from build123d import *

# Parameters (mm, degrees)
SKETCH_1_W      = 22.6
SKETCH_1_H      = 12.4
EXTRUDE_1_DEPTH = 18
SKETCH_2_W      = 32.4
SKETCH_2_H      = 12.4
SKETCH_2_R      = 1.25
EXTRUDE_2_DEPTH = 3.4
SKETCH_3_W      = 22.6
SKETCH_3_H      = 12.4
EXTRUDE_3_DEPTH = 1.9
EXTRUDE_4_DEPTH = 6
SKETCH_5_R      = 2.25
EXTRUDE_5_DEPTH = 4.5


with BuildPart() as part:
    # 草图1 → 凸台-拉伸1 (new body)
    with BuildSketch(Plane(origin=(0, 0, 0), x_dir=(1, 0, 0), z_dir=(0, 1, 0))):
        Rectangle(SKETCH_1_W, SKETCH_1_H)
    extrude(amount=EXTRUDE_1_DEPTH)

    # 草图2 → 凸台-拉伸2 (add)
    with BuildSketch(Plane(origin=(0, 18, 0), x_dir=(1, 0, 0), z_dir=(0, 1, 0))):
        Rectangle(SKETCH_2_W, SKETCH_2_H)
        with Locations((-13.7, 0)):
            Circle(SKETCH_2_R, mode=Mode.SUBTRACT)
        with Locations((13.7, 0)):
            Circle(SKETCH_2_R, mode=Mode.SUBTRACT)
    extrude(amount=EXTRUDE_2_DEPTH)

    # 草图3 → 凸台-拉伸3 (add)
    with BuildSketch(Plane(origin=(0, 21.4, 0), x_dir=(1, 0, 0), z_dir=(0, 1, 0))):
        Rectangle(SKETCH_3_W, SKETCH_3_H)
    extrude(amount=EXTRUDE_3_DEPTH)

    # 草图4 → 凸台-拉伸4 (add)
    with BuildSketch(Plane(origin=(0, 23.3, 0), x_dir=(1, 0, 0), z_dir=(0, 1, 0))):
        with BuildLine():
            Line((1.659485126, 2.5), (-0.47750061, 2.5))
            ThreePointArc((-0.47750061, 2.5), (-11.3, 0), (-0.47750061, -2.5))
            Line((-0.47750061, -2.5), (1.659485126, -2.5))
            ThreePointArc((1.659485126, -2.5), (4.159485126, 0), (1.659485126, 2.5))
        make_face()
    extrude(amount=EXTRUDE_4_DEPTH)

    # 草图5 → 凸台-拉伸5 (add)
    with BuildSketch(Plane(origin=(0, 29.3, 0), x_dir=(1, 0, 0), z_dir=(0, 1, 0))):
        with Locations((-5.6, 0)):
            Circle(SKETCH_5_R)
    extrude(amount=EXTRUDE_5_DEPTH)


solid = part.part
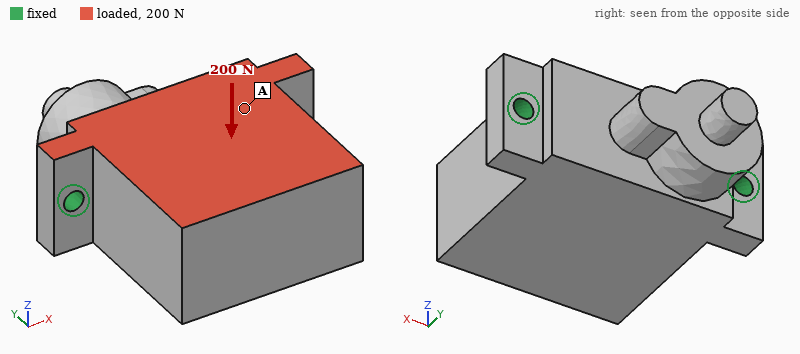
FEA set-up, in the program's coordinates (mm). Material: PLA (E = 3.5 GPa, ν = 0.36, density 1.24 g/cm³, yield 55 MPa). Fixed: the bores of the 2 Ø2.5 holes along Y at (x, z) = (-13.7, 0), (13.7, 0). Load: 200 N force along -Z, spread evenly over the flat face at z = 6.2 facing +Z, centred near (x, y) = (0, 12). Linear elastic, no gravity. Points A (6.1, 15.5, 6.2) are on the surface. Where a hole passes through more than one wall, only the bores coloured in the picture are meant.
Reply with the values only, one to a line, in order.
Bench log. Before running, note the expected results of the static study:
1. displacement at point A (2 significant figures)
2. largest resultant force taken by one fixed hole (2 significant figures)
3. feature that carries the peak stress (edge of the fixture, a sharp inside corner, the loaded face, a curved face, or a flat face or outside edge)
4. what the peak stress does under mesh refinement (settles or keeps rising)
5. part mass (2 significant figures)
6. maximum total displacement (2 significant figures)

0.11 mm
100 N
edge of the fixture
keeps rising
9.6 g
0.30 mm
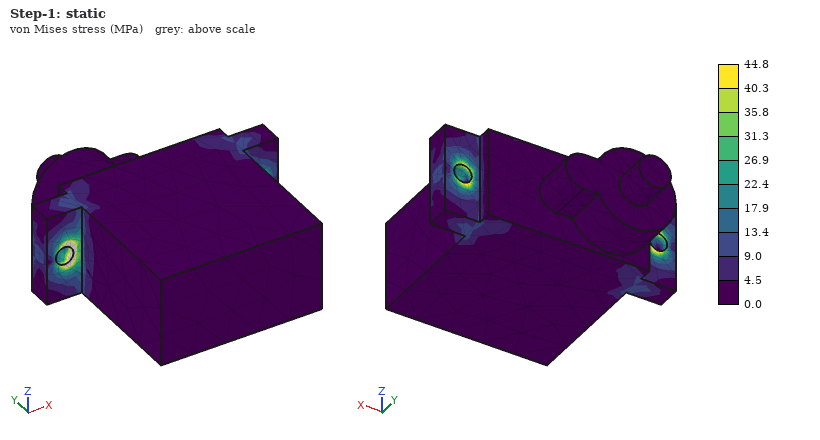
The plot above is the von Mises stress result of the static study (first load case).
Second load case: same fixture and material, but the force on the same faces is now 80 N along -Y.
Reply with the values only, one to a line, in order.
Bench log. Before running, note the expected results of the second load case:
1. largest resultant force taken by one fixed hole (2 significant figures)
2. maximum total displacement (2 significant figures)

40 N
94 µm
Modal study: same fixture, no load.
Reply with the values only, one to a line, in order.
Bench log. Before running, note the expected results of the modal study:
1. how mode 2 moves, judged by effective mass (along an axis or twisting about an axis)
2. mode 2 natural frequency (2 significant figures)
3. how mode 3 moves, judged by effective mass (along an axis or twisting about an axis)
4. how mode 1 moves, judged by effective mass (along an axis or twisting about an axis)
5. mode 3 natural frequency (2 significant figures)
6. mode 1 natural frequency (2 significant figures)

along X
5700 Hz
along Y
along Z
6000 Hz
1600 Hz
